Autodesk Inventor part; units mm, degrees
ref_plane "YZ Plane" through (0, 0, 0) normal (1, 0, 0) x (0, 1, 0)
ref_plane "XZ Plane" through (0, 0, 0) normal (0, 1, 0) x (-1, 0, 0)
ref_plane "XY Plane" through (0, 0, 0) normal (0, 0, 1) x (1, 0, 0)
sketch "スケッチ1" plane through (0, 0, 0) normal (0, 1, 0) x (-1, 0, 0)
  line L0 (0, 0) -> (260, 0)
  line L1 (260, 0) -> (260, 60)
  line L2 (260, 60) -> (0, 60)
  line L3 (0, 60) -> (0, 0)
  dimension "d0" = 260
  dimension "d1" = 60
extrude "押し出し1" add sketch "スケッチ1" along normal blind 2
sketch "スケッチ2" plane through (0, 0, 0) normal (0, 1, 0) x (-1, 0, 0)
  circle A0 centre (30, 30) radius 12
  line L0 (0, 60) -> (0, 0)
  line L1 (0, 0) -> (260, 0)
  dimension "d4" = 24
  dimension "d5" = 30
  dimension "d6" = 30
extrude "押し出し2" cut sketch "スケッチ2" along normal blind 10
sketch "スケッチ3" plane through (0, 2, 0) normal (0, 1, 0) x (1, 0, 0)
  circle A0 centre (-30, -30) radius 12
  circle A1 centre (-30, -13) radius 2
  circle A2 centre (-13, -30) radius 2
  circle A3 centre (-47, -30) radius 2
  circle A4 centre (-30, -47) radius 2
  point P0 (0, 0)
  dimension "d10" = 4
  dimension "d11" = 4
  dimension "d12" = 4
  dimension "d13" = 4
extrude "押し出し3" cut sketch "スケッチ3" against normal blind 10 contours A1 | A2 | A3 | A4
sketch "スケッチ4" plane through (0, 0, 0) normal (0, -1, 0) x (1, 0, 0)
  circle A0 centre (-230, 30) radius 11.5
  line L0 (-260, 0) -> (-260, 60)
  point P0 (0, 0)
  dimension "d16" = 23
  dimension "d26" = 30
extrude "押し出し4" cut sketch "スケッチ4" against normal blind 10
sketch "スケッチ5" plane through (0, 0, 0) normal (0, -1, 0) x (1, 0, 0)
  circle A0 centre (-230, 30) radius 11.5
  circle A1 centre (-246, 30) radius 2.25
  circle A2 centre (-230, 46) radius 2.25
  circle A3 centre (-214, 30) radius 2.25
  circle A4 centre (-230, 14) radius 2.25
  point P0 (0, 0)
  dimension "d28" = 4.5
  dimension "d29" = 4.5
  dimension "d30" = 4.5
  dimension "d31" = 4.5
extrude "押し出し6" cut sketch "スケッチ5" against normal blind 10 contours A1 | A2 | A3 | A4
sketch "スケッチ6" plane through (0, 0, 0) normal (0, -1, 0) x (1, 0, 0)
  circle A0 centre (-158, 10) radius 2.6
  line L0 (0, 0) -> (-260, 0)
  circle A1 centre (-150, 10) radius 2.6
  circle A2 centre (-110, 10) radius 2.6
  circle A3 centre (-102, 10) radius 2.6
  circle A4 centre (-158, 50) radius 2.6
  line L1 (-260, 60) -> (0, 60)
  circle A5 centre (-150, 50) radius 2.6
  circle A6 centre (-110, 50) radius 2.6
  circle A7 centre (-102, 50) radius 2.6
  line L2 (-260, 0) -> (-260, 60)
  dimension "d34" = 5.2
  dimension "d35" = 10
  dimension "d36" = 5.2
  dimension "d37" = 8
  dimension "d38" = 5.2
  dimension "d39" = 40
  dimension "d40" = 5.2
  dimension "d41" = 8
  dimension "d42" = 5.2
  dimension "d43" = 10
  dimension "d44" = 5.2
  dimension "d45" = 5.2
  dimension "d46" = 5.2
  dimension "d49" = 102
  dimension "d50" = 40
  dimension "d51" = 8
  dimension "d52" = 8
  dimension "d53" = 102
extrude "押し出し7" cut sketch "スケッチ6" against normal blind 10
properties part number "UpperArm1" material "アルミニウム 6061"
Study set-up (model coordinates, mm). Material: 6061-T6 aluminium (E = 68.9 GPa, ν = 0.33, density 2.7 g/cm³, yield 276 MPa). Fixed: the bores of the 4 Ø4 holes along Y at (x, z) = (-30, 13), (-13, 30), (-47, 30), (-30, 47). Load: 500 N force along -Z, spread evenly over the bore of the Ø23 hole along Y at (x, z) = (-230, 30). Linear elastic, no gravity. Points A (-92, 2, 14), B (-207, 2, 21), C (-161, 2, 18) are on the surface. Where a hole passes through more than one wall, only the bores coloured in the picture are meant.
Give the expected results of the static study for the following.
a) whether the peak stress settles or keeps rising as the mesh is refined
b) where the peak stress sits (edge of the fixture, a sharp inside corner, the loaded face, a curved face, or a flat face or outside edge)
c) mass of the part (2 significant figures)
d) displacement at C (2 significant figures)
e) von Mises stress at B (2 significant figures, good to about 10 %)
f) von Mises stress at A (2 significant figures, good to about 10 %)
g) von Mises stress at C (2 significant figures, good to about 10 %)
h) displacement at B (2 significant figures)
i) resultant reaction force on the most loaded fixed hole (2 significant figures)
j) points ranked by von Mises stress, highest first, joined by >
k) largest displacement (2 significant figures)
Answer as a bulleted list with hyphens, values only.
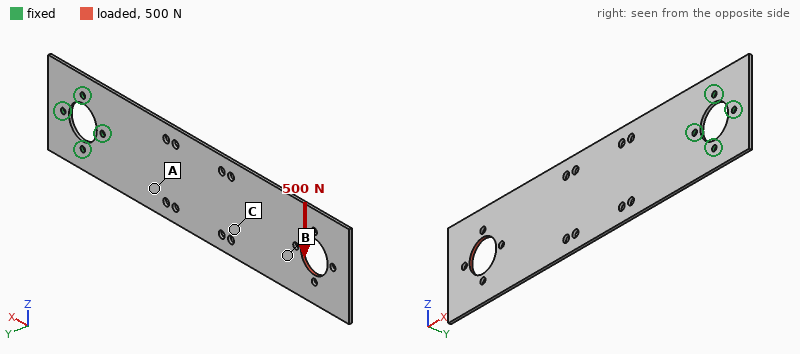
- keeps rising
- edge of the fixture
- 78 g
- 0.33 mm
- 9.5 MPa
- 32 MPa
- 17 MPa
- 0.53 mm
- 2.0 kN
- A > C > B
- 0.79 mm
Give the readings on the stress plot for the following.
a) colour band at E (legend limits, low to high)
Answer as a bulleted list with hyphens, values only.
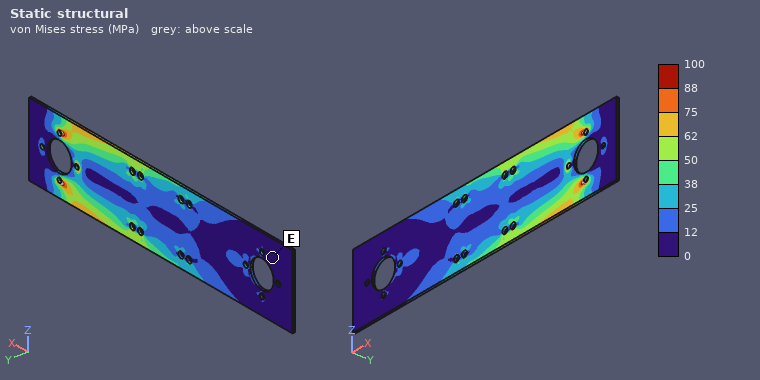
- 0 to 12 MPa
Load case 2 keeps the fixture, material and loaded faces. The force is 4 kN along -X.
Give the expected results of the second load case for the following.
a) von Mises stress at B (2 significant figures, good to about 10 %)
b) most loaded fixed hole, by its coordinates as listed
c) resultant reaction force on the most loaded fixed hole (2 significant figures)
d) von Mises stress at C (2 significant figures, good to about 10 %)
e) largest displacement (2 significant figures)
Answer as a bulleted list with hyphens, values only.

- 40 MPa
- (-47, 30)
- 1.8 kN
- 37 MPa
- 0.12 mm
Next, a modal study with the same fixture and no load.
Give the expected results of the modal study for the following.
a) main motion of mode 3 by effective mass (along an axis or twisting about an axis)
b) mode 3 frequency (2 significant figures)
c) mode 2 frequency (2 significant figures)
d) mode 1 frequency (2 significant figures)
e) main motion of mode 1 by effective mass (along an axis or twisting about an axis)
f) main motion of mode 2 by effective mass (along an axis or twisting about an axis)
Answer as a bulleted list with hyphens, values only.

- twisting about X
- 240 Hz
- 220 Hz
- 37 Hz
- along Y
- along Y
